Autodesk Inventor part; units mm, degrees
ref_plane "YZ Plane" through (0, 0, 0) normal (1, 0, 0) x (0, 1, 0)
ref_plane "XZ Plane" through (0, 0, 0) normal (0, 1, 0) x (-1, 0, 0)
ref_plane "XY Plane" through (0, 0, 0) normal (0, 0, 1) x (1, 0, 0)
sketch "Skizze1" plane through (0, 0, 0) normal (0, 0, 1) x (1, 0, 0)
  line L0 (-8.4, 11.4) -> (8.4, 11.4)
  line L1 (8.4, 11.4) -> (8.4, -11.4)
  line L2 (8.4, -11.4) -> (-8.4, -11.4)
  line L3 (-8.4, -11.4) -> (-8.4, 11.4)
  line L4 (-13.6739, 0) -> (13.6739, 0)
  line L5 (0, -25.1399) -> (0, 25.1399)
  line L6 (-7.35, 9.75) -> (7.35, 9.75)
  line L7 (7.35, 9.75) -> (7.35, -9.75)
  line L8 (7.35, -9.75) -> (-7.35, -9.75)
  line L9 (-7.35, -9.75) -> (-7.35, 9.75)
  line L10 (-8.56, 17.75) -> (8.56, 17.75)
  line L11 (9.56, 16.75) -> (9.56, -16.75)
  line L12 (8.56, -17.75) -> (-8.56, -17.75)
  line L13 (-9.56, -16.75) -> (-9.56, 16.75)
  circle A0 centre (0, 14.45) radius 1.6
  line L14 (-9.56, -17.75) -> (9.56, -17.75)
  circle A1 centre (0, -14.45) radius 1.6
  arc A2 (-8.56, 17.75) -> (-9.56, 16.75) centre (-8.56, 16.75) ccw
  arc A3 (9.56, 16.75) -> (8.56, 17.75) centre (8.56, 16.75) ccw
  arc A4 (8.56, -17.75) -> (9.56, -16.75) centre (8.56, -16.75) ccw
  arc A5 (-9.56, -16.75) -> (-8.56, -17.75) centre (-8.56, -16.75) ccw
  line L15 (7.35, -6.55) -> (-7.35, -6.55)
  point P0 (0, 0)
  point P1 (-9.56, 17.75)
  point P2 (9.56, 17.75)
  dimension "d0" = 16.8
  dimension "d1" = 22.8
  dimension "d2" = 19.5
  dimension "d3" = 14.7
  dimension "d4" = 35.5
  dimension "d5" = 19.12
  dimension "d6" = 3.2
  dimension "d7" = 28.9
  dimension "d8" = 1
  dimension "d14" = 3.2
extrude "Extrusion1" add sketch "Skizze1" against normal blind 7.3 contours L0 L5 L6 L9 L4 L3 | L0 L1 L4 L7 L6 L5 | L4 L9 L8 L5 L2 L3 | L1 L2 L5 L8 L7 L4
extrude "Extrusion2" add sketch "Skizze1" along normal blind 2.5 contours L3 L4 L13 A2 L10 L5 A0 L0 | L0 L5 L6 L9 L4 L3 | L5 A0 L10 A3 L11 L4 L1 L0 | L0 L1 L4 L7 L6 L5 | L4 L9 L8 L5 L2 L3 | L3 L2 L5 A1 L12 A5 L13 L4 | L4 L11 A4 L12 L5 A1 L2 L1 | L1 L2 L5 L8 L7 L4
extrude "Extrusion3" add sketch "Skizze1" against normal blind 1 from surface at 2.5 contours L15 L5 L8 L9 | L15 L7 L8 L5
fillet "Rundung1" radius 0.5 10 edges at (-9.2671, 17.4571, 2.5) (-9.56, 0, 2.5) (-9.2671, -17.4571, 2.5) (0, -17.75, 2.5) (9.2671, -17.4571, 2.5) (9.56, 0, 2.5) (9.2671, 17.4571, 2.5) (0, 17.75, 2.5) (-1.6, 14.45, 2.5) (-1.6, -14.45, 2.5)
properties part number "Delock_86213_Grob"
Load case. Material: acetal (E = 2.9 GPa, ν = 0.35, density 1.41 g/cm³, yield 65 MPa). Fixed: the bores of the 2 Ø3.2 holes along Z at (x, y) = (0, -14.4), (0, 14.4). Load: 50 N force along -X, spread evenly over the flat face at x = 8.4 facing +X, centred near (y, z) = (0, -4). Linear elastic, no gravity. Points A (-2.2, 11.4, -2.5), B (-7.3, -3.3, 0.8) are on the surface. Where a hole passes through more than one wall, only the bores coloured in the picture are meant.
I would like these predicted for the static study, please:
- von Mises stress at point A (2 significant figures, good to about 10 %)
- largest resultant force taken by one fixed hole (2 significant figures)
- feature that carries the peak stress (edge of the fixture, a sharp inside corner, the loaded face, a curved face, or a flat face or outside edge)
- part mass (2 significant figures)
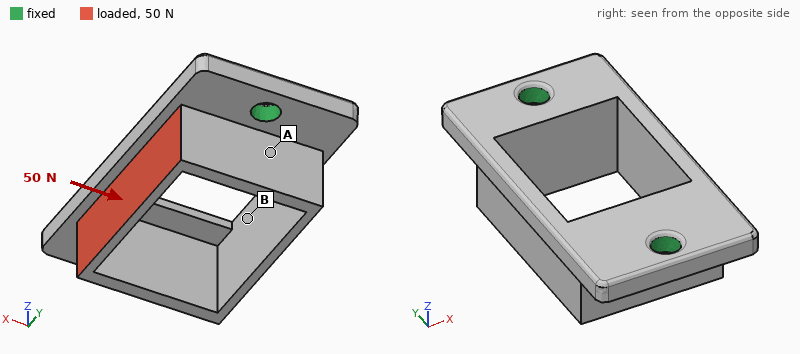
3.8 MPa
28 N
the loaded face
2.4 g
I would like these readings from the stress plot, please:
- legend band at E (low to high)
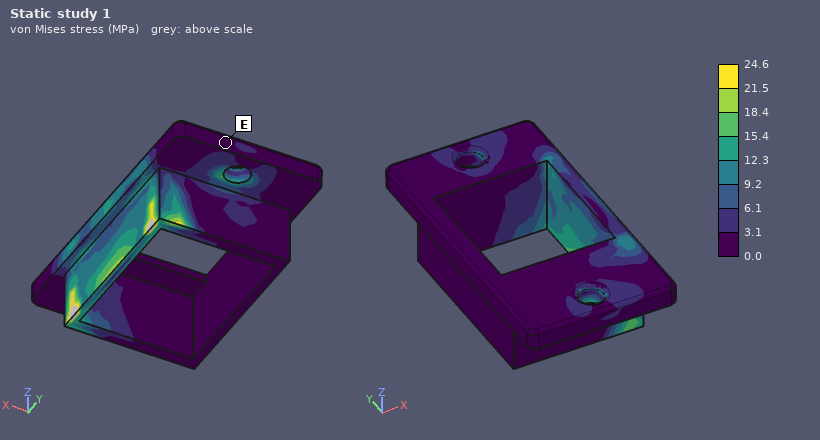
0.0 to 3.1 MPa
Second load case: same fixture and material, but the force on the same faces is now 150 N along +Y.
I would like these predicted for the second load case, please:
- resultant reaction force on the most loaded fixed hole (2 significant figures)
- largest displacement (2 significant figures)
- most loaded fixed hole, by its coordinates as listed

87 N
0.19 mm
(0, -14.4)
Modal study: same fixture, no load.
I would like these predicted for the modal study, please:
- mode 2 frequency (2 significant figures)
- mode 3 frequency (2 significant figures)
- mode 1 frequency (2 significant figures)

4500 Hz
4700 Hz
3100 Hz
